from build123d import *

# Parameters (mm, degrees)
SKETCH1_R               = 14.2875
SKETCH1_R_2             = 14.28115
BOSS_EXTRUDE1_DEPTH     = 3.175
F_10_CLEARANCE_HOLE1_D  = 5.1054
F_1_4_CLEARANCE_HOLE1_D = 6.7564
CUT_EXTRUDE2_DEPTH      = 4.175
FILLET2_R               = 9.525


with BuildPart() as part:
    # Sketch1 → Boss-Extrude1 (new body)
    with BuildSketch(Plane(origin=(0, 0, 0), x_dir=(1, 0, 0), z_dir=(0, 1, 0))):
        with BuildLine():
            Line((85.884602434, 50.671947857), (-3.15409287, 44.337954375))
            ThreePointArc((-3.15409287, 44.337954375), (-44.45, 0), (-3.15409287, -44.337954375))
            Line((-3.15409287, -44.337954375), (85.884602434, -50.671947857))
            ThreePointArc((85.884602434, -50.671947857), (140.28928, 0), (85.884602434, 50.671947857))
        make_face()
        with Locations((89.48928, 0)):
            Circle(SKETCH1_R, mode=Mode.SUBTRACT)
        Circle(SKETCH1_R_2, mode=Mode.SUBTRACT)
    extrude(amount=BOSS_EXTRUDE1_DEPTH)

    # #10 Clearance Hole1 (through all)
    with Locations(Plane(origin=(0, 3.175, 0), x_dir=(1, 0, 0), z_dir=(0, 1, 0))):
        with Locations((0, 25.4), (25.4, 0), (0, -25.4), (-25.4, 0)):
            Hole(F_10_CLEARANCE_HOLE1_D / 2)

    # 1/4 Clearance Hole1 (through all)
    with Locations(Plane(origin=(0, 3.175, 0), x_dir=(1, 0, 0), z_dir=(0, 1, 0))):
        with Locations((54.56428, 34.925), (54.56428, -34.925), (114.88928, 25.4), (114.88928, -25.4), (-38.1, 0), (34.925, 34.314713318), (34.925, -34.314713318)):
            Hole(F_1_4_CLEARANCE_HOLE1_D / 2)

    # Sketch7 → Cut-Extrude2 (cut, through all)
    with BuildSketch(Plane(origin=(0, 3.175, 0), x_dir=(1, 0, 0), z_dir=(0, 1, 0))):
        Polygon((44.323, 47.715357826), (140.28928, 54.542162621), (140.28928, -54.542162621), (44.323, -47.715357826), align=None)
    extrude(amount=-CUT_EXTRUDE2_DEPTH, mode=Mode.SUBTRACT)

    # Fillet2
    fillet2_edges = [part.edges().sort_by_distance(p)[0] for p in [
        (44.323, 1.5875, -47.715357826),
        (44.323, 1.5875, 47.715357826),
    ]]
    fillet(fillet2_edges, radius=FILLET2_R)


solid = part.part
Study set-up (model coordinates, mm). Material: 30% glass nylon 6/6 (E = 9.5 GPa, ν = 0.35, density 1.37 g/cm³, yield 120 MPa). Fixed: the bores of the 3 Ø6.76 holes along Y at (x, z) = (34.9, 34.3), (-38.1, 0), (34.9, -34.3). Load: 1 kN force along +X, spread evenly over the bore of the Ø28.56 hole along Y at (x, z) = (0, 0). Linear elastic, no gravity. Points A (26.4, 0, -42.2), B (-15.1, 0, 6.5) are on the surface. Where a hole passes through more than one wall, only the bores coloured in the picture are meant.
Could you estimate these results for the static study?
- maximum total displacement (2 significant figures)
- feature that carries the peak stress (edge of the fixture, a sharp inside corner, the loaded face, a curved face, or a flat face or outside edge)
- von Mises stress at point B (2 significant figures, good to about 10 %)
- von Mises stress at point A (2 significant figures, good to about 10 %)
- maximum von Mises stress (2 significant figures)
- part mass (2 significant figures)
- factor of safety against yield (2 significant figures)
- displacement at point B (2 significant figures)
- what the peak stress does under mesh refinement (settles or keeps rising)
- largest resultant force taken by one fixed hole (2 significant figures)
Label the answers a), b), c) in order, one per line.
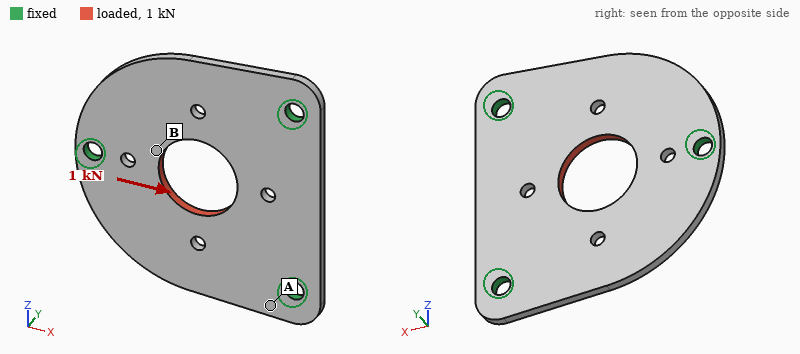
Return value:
a) 28 µm
b) a curved face
c) 5.7 MPa
d) 1.8 MPa
e) 17 MPa
f) 27 g
g) 7.2
h) 15 µm
i) settles
j) 360 N
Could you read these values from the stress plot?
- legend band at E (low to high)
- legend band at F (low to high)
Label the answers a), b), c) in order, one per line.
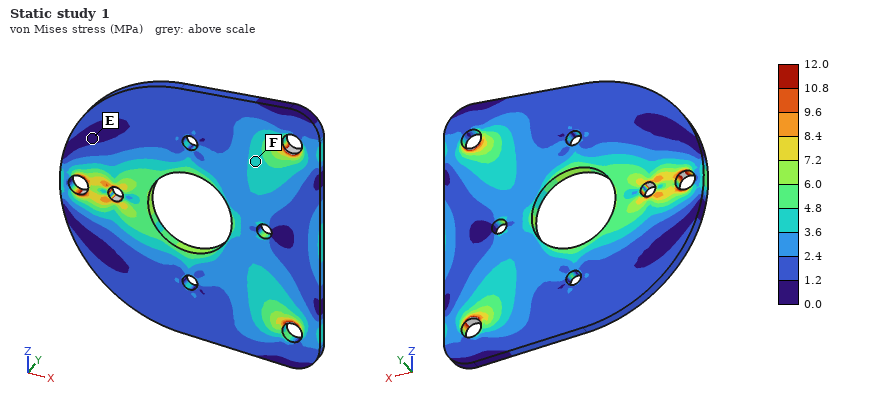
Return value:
a) 0.0 to 1.2 MPa
b) 3.6 to 4.8 MPa
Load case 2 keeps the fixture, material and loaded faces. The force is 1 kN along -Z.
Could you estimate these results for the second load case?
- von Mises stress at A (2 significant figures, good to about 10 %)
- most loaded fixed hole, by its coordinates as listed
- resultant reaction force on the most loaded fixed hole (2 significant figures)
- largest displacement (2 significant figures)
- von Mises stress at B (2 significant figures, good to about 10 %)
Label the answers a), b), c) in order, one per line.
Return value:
a) 1.9 MPa
b) (-38.1, 0)
c) 430 N
d) 31 µm
e) 3.8 MPa
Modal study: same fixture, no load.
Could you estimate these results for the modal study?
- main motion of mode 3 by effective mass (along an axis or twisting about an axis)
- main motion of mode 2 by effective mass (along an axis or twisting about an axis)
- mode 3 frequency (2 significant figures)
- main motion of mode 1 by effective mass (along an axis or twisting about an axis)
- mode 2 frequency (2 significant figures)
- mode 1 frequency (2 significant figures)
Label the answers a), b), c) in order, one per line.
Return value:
a) along Y
b) along Y
c) 1700 Hz
d) twisting about X
e) 1100 Hz
f) 1100 Hz
